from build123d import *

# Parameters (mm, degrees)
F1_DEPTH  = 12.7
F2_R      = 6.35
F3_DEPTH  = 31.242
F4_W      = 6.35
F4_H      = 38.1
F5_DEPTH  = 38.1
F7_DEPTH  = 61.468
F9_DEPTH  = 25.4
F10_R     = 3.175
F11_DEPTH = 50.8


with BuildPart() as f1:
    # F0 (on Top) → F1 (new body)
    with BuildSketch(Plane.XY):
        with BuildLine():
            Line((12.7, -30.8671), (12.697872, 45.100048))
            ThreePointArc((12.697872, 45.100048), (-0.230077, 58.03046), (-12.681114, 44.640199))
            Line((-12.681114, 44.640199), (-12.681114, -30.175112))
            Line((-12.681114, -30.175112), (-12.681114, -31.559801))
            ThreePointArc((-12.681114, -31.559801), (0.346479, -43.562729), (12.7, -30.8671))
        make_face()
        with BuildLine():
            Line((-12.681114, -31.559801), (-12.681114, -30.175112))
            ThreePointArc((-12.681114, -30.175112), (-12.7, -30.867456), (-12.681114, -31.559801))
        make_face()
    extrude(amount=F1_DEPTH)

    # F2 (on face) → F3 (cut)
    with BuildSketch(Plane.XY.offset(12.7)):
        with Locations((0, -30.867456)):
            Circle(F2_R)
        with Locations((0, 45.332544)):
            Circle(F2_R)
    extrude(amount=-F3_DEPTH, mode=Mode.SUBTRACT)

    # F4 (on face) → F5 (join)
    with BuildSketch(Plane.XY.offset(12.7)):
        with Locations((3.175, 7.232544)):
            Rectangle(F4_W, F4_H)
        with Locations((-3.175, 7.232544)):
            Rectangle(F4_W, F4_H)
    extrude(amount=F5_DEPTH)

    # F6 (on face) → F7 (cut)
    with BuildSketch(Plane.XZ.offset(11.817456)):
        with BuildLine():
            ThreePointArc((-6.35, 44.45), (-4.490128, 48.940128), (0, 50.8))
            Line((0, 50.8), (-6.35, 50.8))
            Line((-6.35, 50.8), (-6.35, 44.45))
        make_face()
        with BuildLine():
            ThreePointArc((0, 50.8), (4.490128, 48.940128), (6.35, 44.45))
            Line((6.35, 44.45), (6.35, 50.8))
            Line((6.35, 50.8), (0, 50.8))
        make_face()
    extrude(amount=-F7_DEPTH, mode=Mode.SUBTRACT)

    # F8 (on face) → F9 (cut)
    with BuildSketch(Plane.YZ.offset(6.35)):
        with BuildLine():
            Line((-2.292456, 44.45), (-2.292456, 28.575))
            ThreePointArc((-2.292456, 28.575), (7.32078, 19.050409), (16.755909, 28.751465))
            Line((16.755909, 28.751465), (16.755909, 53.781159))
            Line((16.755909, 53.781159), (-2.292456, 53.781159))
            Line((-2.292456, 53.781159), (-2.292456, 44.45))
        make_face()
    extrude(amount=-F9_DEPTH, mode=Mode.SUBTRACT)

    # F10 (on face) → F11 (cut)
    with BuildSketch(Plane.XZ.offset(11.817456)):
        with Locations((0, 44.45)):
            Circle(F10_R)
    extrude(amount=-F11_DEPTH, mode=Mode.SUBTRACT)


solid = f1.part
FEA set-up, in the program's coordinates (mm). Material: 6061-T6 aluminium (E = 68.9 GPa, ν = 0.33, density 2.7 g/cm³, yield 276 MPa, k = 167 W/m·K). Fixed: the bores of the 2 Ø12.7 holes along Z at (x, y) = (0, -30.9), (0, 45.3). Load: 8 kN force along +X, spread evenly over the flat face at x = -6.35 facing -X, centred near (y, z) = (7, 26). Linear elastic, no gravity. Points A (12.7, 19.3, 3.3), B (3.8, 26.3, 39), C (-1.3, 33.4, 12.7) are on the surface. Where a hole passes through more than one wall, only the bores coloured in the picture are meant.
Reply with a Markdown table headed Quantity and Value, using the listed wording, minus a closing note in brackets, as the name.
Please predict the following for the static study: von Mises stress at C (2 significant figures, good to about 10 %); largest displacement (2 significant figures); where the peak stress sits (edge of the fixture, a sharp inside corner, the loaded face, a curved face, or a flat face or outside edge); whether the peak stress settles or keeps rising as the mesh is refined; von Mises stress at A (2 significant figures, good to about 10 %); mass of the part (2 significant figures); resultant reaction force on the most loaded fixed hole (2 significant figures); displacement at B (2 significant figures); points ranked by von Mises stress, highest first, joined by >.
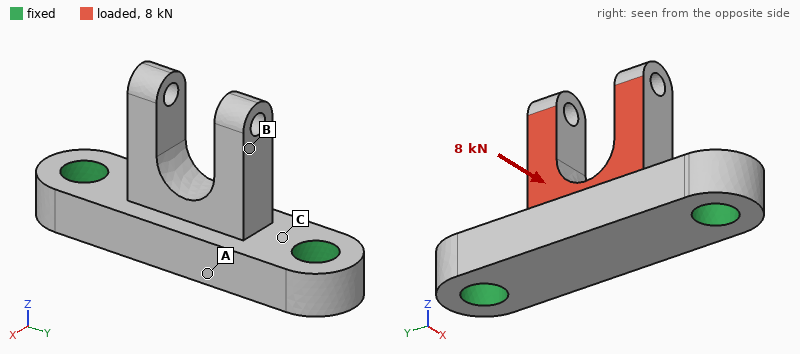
| Quantity | Value |
|---|---|
| von Mises stress at C | 130 MPa |
| largest displacement | 0.37 mm |
| where the peak stress sits | edge of the fixture |
| whether the peak stress settles or keeps rising as the mesh is refined | keeps rising |
| von Mises stress at A | 49 MPa |
| mass of the part | 100 g |
| resultant reaction force on the most loaded fixed hole | 4.0 kN |
| displacement at B | 0.26 mm |
| points ranked by von Mises stress, highest first, joined by > | C > A > B |
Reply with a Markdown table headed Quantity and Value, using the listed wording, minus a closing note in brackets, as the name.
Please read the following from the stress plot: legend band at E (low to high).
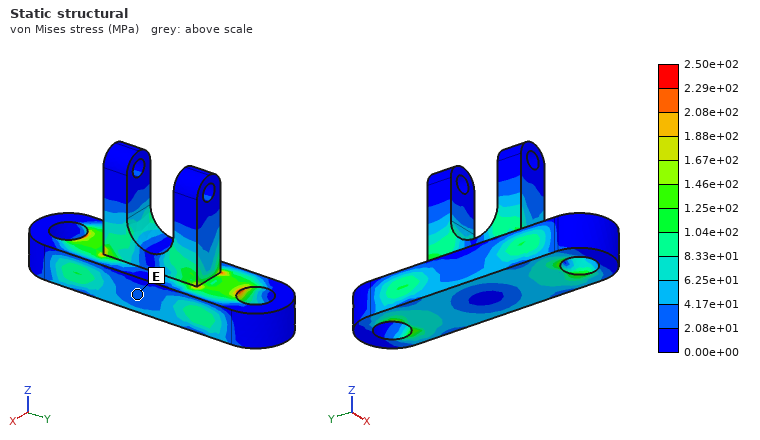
| Quantity | Value |
|---|---|
| legend band at E | 2.08e+01 to 4.17e+01 MPa |
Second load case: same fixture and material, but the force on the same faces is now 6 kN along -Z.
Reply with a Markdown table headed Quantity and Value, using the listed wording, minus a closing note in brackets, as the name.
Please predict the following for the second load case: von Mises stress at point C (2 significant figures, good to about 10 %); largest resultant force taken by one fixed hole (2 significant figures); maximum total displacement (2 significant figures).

| Quantity | Value |
|---|---|
| von Mises stress at point C | 32 MPa |
| largest resultant force taken by one fixed hole | 3.1 kN |
| maximum total displacement | 0.11 mm |
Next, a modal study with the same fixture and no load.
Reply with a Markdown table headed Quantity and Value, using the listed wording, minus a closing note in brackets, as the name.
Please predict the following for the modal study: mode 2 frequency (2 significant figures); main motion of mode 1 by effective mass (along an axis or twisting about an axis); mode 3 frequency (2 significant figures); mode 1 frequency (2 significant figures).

| Quantity | Value |
|---|---|
| mode 2 frequency | 7400 Hz |
| main motion of mode 1 by effective mass | along X |
| mode 3 frequency | 7900 Hz |
| mode 1 frequency | 5300 Hz |
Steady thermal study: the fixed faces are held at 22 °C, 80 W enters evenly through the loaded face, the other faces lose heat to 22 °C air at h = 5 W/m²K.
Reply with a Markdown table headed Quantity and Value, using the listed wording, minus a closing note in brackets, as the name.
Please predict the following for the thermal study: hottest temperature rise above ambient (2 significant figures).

| Quantity | Value |
|---|---|
| hottest temperature rise above ambient | 41 K |
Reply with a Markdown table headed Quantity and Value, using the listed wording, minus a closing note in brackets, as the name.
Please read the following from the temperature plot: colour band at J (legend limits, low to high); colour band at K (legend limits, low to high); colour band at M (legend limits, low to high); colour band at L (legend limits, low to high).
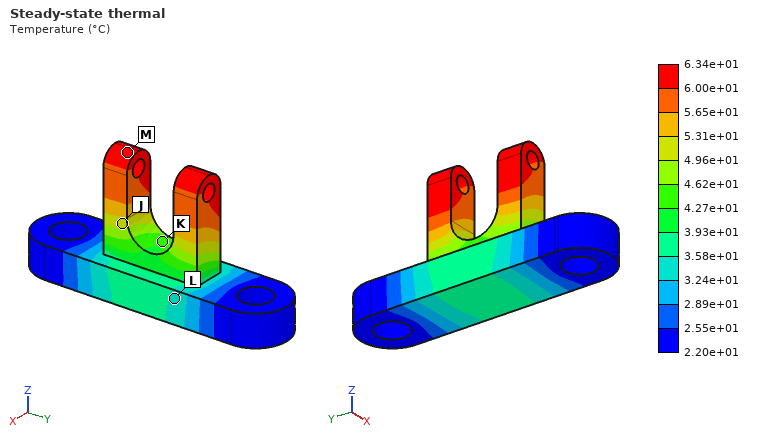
| Quantity | Value |
|---|---|
| colour band at J | 4.96e+01 to 5.31e+01 °C |
| colour band at K | 4.27e+01 to 4.62e+01 °C |
| colour band at M | 6.00e+01 to 6.34e+01 °C |
| colour band at L | 3.24e+01 to 3.58e+01 °C |
